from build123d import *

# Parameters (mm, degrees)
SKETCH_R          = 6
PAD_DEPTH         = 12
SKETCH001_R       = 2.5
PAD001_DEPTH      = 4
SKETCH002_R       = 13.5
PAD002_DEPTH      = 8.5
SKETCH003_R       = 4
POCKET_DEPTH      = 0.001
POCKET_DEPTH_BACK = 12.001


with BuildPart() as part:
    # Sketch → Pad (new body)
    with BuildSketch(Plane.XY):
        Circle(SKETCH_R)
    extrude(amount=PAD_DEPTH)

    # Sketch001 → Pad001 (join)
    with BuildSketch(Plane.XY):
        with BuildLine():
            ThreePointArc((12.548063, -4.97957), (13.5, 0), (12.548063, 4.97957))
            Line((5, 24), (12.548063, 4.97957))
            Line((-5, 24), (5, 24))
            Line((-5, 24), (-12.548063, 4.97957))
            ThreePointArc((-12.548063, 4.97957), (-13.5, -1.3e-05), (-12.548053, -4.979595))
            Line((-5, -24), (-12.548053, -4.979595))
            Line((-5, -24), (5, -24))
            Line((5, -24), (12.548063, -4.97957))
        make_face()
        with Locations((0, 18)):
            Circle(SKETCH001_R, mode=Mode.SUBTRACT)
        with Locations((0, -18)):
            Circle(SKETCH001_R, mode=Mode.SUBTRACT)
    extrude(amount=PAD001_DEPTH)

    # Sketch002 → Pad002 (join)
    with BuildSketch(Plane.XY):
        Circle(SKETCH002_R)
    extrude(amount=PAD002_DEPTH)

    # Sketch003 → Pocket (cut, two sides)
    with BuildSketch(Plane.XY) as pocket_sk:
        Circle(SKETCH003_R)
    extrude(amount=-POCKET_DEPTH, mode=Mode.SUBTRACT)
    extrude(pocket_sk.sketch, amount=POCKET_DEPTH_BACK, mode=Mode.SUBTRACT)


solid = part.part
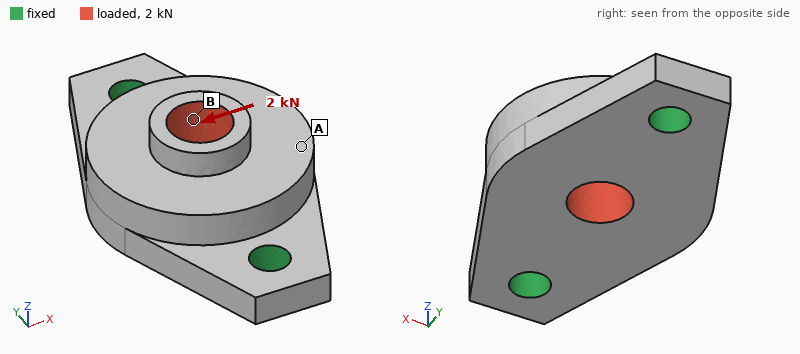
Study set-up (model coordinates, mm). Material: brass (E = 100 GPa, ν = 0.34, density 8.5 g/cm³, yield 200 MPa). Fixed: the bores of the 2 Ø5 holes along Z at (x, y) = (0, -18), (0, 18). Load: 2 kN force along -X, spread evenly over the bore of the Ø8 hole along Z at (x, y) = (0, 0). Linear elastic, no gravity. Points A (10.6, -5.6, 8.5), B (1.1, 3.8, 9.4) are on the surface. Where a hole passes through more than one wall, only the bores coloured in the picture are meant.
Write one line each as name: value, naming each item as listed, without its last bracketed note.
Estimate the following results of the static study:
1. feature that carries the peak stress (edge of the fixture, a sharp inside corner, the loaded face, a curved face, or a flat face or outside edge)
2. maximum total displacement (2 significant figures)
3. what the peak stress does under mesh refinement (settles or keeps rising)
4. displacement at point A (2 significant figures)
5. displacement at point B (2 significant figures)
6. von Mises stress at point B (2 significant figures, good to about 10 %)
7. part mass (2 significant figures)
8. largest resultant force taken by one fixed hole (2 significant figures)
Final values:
feature that carries the peak stress: edge of the fixture
maximum total displacement: 25 µm
what the peak stress does under mesh refinement: keeps rising
displacement at point A: 21 µm
displacement at point B: 16 µm
von Mises stress at point B: 25 MPa
part mass: 50 g
largest resultant force taken by one fixed hole: 1.0 kN
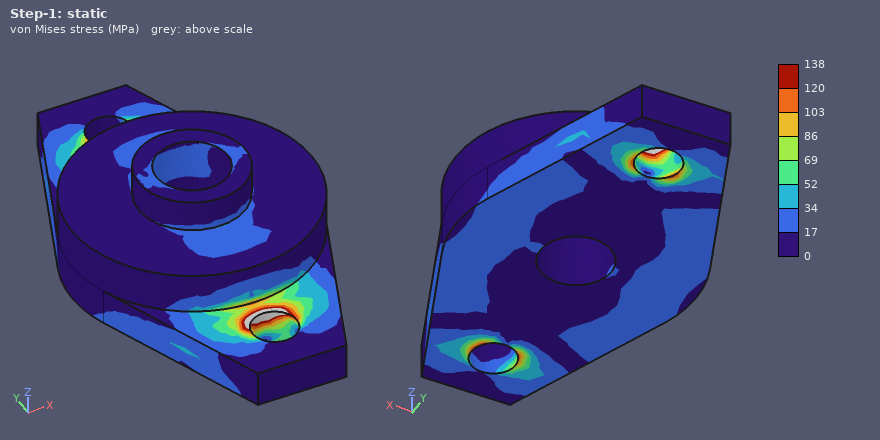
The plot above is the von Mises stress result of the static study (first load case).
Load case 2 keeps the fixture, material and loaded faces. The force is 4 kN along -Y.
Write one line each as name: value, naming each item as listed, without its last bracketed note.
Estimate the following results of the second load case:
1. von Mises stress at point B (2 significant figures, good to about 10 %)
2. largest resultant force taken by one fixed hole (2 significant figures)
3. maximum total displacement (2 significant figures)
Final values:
von Mises stress at point B: 27 MPa
largest resultant force taken by one fixed hole: 2.1 kN
maximum total displacement: 8.8 µm
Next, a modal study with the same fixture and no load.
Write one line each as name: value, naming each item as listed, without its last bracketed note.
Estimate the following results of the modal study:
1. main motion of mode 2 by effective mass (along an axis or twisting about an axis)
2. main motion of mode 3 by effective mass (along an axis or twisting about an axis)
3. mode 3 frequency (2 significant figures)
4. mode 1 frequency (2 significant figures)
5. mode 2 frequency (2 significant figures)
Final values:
main motion of mode 2 by effective mass: along Z
main motion of mode 3 by effective mass: along X
mode 3 frequency: 19 kHz
mode 1 frequency: 7200 Hz
mode 2 frequency: 11 kHz
